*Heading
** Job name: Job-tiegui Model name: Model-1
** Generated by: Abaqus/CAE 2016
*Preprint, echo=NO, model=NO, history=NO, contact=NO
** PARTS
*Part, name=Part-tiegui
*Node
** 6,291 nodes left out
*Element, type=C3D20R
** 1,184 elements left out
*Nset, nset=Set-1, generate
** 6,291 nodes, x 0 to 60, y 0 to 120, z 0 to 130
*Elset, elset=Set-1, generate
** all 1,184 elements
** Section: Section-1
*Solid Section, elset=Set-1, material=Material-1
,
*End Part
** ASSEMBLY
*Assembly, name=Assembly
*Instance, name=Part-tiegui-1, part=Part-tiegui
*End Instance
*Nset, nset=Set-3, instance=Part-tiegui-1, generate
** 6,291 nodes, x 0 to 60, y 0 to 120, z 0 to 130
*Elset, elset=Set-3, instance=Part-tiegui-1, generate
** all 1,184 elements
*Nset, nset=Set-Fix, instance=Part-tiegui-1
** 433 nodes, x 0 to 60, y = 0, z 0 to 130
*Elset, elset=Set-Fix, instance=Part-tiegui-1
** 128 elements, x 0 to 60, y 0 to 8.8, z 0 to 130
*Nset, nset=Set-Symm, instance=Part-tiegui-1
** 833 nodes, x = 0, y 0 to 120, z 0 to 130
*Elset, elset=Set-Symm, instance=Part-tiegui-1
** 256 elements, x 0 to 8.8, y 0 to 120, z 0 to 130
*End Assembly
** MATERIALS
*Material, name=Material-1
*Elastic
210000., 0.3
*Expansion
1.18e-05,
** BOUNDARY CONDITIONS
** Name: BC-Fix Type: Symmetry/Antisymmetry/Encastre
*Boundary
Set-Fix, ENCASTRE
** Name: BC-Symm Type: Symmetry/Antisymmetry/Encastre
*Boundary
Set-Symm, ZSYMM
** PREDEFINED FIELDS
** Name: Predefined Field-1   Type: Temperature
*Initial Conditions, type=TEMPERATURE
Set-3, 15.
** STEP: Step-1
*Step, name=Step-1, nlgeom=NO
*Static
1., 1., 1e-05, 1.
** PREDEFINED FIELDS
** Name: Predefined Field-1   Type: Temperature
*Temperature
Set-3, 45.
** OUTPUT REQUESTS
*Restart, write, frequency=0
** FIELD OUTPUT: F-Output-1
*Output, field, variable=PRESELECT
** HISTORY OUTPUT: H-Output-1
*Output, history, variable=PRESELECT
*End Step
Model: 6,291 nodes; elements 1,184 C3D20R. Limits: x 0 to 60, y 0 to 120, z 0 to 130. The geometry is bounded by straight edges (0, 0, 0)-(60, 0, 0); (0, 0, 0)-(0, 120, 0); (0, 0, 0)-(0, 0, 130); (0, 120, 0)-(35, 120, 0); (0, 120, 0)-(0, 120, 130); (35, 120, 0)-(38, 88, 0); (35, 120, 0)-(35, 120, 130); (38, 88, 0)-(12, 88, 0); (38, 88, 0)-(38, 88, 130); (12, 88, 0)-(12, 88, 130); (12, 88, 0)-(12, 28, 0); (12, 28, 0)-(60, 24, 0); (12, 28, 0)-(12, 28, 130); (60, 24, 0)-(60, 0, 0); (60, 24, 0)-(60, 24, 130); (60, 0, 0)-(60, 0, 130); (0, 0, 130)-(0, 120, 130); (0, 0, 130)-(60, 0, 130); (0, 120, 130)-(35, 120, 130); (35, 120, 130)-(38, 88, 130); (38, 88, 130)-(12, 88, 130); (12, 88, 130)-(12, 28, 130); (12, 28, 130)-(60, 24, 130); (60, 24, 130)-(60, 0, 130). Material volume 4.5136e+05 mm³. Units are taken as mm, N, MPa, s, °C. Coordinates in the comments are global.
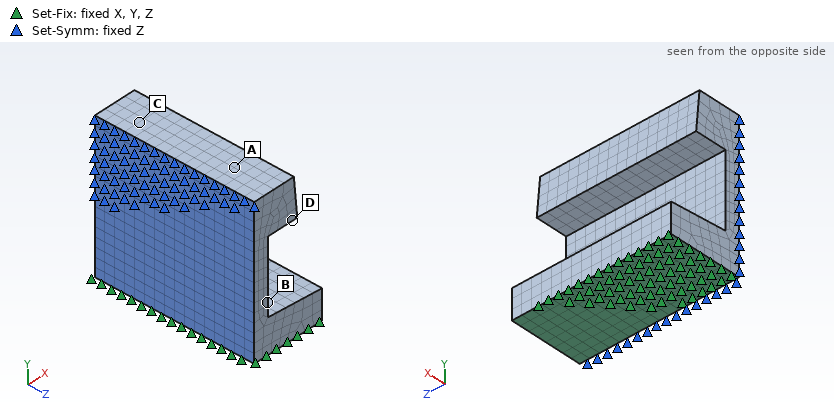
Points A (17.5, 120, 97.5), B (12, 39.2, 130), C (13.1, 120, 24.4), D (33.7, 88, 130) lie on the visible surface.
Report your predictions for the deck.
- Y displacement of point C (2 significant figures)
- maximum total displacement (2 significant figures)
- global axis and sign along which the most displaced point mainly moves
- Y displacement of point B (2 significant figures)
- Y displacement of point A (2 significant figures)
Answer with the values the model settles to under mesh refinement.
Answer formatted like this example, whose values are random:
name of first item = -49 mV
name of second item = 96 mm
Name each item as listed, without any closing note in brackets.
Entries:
Y displacement of point C = 0.048 mm
maximum total displacement = 0.057 mm
global axis and sign along which the most displaced point mainly moves = +Y
Y displacement of point B = 0.018 mm
Y displacement of point A = 0.047 mm
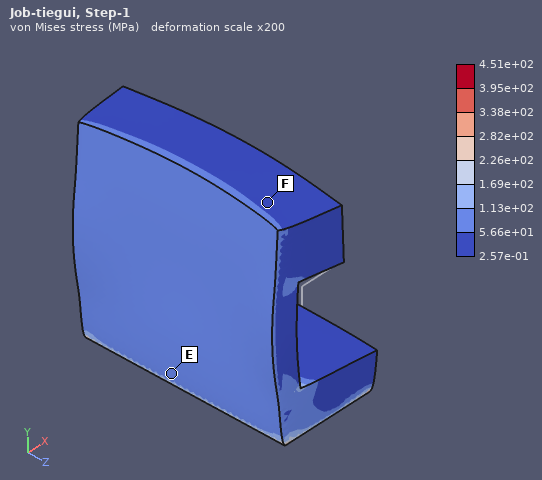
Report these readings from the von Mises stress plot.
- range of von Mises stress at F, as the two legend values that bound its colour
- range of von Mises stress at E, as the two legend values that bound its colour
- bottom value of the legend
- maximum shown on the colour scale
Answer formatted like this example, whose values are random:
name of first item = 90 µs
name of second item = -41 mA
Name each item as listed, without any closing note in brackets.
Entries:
range of von Mises stress at F, as the two legend values that bound its colour = 2.57e-01 to 5.66e+01 MPa
range of von Mises stress at E, as the two legend values that bound its colour = 5.66e+01 to 1.13e+02 MPa
bottom value of the legend = 2.57e-01 MPa
maximum shown on the colour scale = 4.51e+02 MPa
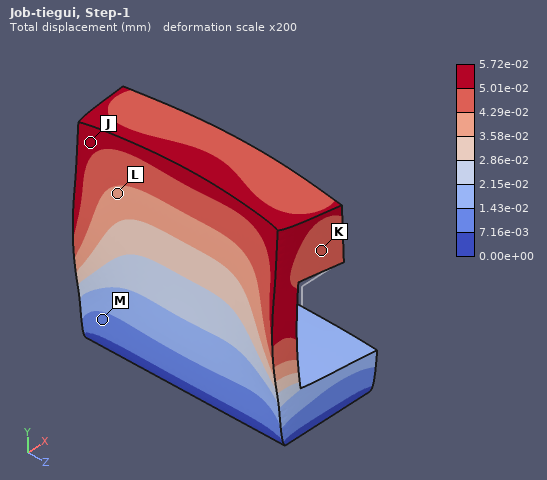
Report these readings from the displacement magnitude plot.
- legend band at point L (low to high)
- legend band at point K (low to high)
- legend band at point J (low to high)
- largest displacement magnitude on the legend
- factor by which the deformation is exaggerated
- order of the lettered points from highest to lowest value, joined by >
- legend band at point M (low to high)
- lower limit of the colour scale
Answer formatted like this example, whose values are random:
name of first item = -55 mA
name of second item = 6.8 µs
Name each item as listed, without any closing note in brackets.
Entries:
legend band at point L = 3.58e-02 to 4.29e-02 mm
legend band at point K = 4.29e-02 to 5.01e-02 mm
legend band at point J = 5.01e-02 to 5.72e-02 mm
largest displacement magnitude on the legend = 5.72e-02 mm
factor by which the deformation is exaggerated = 200
order of the lettered points from highest to lowest value, joined by > = J > K > L > M
legend band at point M = 7.16e-03 to 1.43e-02 mm
lower limit of the colour scale = 0.00e+00 mm
